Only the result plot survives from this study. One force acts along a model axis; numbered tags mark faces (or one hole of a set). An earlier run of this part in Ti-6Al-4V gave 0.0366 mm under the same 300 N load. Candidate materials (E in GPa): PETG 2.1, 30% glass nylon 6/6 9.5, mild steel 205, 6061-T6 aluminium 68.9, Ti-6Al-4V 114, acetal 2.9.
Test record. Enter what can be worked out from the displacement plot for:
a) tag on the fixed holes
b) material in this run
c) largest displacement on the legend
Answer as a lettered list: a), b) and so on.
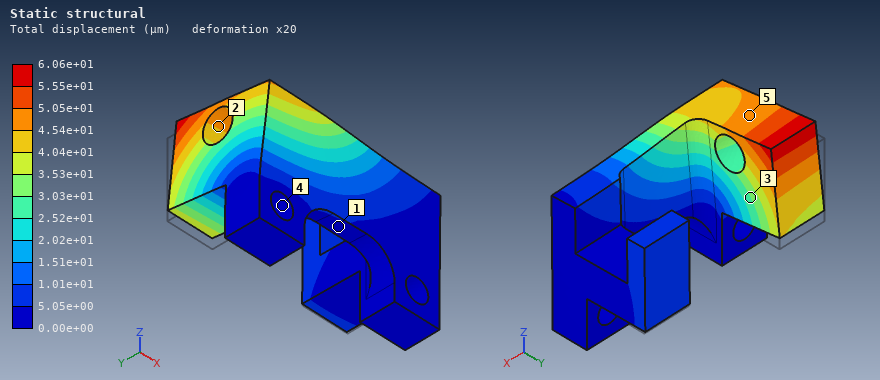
a) 4
b) 6061-T6 aluminium
c) 6.06e+01 µm
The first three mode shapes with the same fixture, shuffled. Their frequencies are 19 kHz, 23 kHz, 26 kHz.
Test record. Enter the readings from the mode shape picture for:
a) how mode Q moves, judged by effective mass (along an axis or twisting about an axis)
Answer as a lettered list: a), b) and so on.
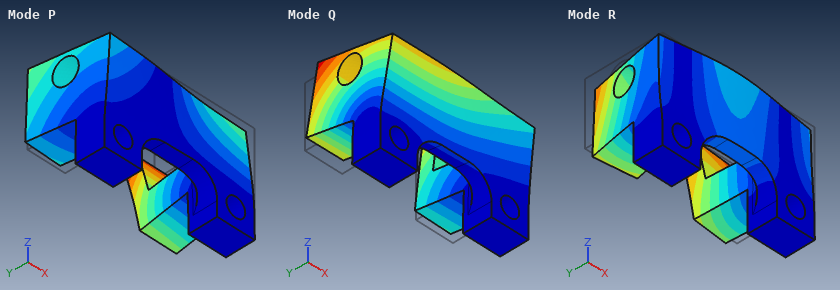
a) along Y
